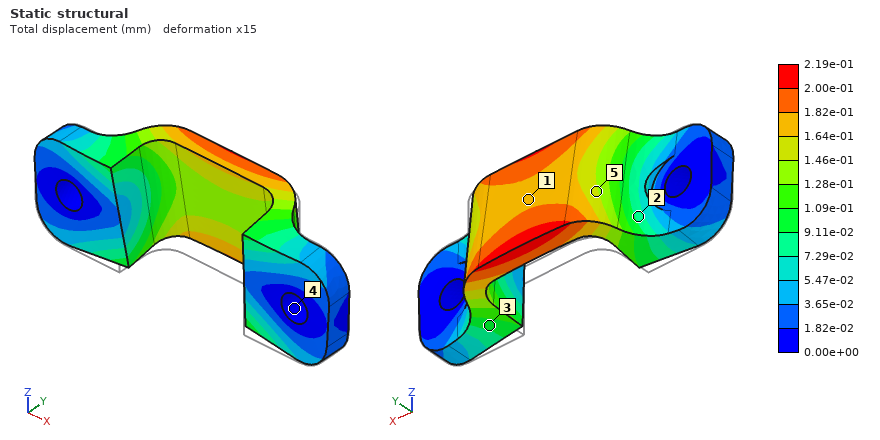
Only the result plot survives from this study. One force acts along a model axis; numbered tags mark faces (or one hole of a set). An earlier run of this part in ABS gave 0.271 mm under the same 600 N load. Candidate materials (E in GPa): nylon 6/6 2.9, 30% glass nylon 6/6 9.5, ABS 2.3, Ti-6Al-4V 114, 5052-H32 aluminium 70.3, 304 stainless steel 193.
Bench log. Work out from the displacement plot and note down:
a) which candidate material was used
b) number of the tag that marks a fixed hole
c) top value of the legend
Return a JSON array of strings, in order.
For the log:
["nylon 6/6", "4", "2.19e-01 mm"]
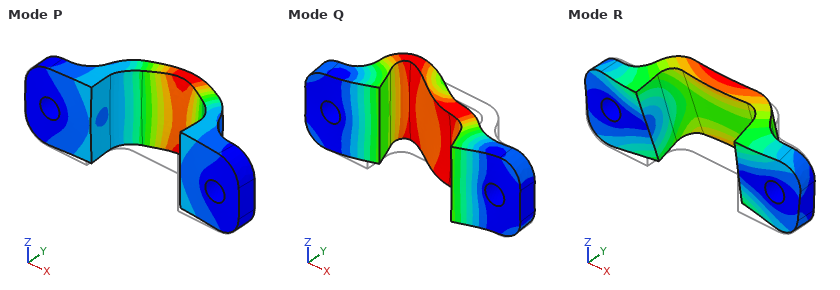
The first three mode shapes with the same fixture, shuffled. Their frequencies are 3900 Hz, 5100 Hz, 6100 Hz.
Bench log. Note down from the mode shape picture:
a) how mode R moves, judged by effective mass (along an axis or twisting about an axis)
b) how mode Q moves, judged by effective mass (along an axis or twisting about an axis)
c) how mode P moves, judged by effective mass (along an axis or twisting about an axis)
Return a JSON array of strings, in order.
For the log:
["along Z", "along X", "along Y"]
